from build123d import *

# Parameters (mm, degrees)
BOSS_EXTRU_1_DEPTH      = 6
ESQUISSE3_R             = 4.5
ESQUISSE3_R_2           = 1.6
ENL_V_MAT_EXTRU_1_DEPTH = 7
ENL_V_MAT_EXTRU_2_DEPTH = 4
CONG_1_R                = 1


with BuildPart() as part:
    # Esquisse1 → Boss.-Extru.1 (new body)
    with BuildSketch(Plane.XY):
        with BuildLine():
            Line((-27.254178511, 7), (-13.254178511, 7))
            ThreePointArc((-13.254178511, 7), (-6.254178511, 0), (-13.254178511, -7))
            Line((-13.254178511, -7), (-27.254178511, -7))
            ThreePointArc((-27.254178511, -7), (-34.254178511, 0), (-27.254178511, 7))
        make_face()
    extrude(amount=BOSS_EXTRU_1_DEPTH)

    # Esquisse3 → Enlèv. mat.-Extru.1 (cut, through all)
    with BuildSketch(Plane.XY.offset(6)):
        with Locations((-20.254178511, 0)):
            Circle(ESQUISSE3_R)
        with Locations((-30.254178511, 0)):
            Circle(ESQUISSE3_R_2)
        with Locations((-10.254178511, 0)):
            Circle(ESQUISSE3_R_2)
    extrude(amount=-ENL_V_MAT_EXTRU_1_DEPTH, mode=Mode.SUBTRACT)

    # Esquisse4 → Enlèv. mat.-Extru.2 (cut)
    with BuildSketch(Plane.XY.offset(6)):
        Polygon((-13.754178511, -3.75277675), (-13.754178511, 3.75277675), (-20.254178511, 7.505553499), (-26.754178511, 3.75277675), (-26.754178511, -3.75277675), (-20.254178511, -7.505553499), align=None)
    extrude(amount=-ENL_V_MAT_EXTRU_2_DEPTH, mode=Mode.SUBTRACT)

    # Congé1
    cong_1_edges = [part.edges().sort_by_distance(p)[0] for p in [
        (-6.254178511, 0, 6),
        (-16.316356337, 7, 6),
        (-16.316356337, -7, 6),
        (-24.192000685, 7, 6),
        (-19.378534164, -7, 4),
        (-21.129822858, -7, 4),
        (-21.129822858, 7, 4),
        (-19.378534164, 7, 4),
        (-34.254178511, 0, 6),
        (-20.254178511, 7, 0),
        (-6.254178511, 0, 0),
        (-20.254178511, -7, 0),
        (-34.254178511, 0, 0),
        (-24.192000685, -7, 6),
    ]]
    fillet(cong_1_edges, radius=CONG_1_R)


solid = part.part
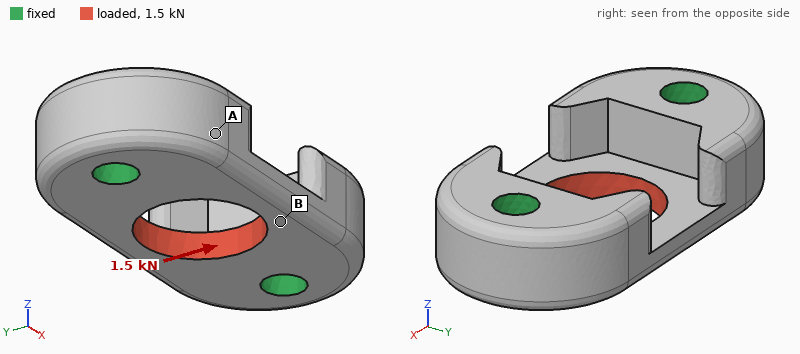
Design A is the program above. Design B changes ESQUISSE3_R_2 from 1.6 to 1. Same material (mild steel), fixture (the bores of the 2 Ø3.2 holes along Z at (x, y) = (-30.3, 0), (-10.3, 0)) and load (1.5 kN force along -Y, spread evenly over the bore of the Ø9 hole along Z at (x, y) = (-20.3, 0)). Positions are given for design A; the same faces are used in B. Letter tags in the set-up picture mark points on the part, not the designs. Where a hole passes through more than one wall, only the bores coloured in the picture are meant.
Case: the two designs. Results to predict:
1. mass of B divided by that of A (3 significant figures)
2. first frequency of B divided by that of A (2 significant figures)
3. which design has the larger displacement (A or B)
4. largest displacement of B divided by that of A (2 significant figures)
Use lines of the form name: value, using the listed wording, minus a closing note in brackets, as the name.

mass of B divided by that of A: 1.05
first frequency of B divided by that of A: 0.85
which design has the larger displacement: B
largest displacement of B divided by that of A: 1.2
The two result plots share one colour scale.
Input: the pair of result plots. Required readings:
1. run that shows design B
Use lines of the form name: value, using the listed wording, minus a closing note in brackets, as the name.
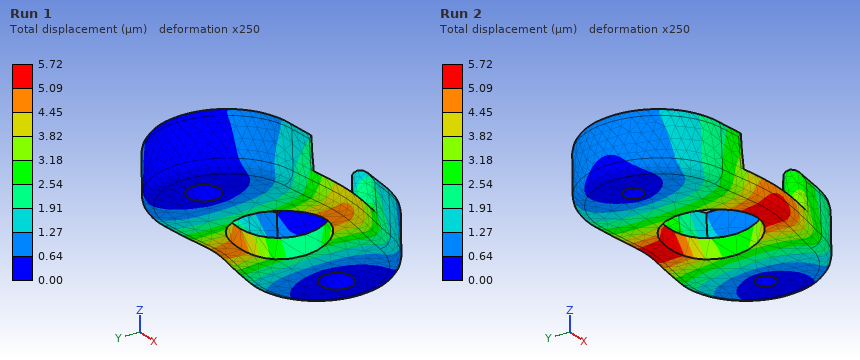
run that shows design B: Run 2
